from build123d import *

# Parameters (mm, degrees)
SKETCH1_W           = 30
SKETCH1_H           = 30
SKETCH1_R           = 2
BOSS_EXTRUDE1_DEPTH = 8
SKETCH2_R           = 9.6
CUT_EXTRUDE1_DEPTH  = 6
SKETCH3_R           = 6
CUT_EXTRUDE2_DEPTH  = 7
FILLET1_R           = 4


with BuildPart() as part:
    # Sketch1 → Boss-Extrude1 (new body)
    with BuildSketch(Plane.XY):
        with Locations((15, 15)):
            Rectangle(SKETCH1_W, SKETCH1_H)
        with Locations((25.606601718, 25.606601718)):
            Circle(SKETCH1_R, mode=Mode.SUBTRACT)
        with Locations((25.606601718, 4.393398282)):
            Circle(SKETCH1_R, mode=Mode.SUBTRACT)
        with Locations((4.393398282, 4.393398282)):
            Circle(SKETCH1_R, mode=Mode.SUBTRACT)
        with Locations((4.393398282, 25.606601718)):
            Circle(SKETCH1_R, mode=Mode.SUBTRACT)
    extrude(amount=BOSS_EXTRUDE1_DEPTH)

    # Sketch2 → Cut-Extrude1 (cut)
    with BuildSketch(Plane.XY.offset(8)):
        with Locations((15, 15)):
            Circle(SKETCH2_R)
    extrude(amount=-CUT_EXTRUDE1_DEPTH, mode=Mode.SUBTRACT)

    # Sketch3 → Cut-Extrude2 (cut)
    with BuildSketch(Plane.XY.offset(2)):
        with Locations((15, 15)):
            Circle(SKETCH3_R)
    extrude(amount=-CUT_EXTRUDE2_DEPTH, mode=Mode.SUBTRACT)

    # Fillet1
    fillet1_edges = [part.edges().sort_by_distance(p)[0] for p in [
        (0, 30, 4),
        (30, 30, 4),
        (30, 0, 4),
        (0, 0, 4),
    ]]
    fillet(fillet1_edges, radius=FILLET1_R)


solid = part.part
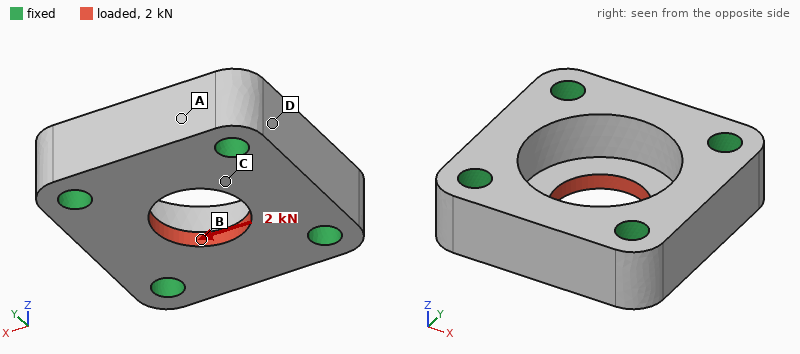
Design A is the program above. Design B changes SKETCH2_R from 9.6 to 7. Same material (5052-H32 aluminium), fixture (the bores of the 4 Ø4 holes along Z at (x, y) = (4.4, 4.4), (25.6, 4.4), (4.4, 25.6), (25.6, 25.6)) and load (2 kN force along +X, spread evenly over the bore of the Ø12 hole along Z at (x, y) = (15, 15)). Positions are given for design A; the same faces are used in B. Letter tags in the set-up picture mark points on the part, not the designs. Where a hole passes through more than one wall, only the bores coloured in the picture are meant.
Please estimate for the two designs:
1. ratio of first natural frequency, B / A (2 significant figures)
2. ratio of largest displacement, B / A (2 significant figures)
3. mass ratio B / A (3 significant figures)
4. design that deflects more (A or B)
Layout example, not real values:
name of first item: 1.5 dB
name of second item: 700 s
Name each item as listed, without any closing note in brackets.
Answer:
ratio of first natural frequency, B / A: 0.97
ratio of largest displacement, B / A: 0.80
mass ratio B / A: 1.17
design that deflects more: A
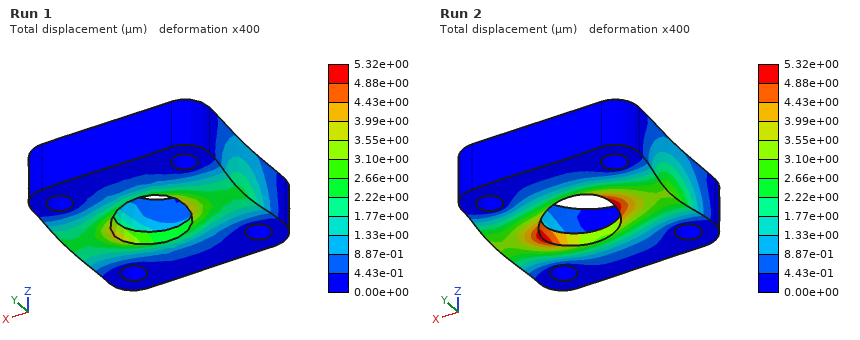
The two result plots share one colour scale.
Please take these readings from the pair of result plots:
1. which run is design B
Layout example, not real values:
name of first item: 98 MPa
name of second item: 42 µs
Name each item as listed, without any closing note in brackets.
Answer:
which run is design B: Run 1
